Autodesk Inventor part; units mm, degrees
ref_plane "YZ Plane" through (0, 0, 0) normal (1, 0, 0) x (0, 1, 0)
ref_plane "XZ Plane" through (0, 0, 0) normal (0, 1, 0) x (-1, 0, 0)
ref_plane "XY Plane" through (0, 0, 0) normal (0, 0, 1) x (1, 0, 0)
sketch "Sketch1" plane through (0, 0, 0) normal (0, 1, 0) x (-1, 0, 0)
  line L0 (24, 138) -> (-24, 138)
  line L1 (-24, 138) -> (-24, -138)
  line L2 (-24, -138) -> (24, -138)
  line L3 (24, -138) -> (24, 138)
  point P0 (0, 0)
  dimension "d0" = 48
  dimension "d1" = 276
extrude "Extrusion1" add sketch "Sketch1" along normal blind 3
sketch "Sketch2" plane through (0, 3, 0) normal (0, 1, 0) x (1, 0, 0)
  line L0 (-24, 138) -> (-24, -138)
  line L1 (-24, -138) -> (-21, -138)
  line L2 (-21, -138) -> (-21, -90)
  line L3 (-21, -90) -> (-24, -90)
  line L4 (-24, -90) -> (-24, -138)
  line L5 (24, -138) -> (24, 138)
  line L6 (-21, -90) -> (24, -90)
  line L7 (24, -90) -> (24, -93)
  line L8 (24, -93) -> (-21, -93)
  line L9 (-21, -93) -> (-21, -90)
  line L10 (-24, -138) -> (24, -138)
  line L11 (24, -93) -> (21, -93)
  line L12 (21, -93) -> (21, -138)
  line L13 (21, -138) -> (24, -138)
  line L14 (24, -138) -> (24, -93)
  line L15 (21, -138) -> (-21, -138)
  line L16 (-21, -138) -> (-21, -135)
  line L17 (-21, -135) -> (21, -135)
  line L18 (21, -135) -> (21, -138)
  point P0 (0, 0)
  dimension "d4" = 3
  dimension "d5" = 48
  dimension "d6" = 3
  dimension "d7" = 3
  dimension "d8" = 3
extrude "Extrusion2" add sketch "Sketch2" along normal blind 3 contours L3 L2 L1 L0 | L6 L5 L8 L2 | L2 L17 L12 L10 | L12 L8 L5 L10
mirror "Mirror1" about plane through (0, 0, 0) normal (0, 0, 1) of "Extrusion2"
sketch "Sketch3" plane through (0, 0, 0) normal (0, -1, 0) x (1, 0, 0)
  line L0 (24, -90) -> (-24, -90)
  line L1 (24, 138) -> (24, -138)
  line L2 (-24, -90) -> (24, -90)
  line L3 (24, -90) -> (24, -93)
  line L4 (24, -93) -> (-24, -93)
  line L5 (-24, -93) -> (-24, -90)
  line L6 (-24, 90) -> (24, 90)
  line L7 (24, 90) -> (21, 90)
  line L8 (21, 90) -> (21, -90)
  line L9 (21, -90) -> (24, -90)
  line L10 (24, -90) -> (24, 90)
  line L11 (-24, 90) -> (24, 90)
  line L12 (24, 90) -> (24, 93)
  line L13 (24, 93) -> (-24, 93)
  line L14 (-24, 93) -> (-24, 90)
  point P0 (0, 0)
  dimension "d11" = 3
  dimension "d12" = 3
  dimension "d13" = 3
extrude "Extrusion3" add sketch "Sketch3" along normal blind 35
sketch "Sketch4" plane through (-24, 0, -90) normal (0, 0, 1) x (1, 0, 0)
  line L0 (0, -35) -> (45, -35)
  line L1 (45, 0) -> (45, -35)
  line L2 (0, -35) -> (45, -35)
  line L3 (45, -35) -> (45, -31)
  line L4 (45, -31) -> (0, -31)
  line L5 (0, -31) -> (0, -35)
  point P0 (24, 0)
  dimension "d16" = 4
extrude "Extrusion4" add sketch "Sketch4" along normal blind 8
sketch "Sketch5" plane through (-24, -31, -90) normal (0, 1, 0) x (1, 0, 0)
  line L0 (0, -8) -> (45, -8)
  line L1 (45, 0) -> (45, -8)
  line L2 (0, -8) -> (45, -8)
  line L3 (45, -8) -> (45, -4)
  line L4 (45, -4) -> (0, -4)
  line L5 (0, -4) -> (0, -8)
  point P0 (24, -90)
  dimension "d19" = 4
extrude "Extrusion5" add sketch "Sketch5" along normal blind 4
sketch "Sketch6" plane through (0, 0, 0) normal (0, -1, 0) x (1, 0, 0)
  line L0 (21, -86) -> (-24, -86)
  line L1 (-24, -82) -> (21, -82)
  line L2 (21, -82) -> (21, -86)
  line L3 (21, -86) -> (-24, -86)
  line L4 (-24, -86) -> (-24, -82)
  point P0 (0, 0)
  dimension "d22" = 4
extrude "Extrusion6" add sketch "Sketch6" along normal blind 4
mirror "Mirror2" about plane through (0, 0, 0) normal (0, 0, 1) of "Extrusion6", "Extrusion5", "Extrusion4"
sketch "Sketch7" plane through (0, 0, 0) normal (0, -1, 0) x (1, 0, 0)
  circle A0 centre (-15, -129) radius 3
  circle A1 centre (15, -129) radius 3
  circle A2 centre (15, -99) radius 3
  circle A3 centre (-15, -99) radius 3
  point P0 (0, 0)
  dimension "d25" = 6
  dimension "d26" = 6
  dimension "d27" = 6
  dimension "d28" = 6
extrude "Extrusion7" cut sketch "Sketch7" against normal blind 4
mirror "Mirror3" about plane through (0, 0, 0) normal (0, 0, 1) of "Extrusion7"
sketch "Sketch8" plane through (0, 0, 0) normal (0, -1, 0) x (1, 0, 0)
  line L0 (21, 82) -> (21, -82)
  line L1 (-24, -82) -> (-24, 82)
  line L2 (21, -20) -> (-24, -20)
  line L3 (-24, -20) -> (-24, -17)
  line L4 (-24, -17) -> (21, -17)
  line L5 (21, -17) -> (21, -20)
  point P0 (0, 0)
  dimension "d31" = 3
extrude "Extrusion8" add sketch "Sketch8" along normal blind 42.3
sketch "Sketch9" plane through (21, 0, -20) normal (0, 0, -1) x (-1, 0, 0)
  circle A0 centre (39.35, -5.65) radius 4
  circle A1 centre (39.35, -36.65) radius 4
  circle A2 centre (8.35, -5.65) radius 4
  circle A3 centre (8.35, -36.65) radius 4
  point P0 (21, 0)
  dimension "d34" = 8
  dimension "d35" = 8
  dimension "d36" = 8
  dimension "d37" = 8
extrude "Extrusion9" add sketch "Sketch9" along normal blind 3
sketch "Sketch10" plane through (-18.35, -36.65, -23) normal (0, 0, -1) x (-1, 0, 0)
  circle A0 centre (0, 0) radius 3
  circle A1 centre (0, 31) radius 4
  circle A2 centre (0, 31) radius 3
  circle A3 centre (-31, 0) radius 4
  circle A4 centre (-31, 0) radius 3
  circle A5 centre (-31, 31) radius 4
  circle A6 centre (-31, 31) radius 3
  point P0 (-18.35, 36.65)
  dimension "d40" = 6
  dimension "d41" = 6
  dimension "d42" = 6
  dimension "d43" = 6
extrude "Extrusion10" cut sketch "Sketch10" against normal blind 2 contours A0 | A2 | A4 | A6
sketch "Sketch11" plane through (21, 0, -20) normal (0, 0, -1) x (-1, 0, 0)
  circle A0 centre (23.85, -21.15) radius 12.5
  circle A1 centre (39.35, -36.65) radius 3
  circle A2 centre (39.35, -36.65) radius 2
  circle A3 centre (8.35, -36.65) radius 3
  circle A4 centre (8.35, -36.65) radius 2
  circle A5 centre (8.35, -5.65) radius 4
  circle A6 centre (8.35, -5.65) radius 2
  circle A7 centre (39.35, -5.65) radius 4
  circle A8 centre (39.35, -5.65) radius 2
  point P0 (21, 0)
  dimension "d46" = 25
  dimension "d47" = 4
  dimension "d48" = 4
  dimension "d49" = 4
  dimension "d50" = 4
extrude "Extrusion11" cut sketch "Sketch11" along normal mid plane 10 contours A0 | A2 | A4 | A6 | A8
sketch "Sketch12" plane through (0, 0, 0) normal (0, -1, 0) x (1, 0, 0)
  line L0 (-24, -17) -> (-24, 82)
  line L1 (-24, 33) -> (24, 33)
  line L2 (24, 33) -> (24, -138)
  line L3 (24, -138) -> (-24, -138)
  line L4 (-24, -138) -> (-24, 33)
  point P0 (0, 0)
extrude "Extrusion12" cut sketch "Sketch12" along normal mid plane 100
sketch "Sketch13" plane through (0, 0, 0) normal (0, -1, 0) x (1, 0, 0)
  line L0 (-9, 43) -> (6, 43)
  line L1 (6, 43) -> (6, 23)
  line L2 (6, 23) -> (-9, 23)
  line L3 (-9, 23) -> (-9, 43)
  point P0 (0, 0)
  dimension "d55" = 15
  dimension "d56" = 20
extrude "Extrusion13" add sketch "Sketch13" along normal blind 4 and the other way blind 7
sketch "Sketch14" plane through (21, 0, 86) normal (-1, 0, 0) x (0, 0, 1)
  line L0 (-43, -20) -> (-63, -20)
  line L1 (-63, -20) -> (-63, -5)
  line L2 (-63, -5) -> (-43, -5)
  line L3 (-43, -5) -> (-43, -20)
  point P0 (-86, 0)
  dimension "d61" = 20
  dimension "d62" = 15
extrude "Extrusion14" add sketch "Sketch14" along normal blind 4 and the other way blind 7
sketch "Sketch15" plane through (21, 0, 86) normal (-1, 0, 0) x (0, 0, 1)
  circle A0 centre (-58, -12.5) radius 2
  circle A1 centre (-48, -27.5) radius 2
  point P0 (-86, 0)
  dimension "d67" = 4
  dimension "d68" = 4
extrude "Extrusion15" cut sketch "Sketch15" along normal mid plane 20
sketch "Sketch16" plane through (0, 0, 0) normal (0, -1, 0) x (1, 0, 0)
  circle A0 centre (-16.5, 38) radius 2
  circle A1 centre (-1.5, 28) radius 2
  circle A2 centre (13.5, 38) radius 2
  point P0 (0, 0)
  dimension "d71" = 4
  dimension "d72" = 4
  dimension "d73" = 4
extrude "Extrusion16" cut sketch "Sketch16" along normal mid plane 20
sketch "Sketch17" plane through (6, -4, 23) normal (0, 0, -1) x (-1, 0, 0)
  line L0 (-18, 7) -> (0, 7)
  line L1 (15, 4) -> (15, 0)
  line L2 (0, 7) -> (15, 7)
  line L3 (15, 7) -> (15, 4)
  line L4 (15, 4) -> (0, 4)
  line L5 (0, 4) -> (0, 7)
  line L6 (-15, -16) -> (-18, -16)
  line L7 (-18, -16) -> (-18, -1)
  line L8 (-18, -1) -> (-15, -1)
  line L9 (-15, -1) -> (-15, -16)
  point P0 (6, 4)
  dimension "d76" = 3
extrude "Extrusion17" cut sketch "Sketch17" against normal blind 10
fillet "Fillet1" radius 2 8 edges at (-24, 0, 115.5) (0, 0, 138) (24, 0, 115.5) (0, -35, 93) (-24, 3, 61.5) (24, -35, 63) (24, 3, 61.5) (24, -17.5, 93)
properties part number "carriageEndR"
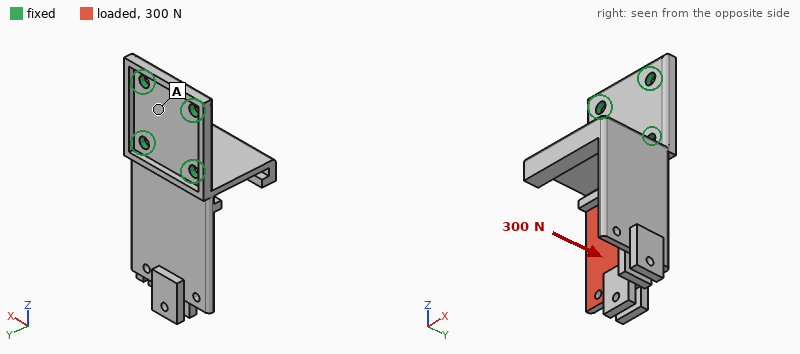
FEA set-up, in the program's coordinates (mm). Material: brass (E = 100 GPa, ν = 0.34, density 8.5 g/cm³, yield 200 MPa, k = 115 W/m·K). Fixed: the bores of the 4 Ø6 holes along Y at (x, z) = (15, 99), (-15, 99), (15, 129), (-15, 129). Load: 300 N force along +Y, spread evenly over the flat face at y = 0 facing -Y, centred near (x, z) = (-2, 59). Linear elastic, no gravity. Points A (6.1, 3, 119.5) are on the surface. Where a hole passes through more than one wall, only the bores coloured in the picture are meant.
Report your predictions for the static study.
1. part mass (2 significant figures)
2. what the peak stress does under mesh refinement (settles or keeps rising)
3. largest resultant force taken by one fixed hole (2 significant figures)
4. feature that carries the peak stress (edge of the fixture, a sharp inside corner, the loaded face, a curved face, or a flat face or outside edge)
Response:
290 g
keeps rising
310 N
edge of the fixture
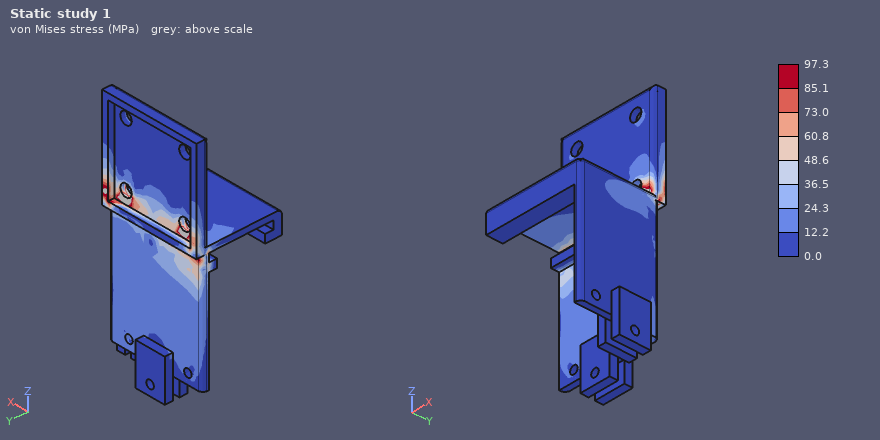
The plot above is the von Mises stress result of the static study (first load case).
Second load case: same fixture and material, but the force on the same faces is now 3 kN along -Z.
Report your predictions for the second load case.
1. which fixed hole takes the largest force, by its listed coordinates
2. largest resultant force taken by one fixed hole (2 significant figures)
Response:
(-15, 99)
1.5 kN
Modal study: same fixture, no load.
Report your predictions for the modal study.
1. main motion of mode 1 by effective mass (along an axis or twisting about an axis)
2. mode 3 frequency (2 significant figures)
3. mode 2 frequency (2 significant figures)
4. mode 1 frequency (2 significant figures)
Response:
along Y
1400 Hz
840 Hz
330 Hz
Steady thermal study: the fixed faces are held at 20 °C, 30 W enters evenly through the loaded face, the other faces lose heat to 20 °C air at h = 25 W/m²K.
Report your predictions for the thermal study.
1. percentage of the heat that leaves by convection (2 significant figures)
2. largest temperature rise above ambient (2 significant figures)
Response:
29 %
45 K
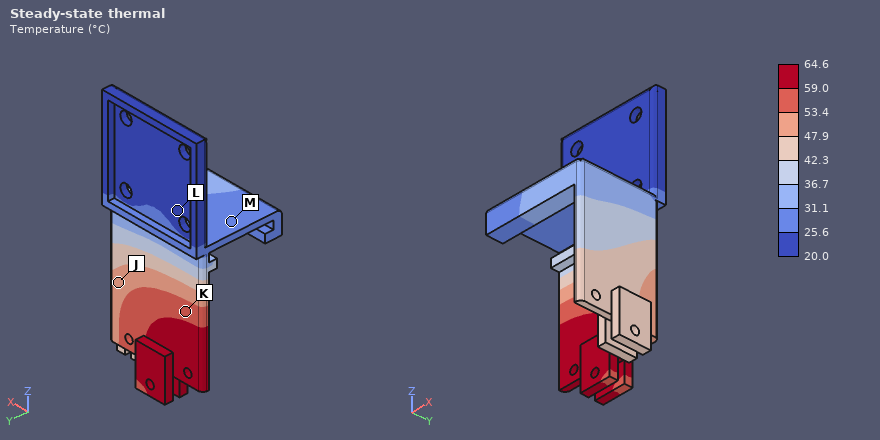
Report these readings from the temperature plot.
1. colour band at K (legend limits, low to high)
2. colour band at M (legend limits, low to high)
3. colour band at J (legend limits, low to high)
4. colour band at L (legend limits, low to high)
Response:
53.4 to 59.0 °C
25.6 to 31.1 °C
47.9 to 53.4 °C
20.0 to 25.6 °C
